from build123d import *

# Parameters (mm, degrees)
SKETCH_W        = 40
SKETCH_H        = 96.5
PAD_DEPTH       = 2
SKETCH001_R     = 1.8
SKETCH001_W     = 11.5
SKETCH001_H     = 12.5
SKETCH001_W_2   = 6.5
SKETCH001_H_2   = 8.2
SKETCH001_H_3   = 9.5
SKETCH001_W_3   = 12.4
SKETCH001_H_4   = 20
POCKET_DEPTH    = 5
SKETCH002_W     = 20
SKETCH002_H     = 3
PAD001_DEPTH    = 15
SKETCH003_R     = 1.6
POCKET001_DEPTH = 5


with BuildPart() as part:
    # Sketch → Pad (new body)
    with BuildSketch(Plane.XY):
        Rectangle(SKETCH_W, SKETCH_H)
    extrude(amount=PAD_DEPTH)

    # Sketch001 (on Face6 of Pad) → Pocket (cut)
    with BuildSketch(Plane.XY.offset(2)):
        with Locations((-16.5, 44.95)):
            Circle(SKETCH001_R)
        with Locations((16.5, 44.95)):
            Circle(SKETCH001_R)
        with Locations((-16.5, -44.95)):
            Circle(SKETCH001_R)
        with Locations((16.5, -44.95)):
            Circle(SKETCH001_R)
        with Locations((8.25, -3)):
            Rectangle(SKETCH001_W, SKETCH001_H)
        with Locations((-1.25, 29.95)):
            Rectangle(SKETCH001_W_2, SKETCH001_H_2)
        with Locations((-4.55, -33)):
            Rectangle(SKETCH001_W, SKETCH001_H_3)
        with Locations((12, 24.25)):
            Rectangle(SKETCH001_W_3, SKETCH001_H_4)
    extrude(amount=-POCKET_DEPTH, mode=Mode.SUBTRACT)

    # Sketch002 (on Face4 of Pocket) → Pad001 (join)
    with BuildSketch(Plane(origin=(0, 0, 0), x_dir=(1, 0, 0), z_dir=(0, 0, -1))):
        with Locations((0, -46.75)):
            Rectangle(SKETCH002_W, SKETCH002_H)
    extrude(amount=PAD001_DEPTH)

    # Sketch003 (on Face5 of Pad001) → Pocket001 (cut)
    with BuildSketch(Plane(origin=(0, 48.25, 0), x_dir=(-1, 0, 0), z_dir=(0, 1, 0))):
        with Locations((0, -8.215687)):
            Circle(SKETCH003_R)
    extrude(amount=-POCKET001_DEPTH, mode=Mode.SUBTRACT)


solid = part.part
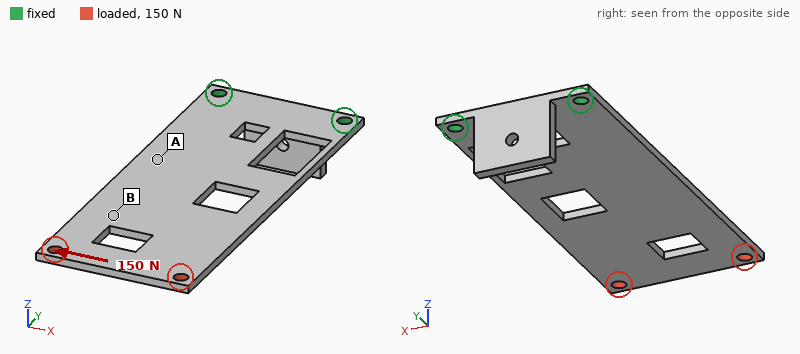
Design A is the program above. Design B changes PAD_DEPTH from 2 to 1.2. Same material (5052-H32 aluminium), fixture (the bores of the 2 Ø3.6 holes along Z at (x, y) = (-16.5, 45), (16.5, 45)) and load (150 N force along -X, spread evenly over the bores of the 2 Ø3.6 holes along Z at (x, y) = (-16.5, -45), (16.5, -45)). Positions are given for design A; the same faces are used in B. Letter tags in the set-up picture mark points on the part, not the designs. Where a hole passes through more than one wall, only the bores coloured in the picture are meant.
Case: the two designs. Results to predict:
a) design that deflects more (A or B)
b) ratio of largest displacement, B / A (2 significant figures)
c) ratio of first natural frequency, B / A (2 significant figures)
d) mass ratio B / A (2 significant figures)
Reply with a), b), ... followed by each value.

a) B
b) 1.7
c) 0.61
d) 0.65
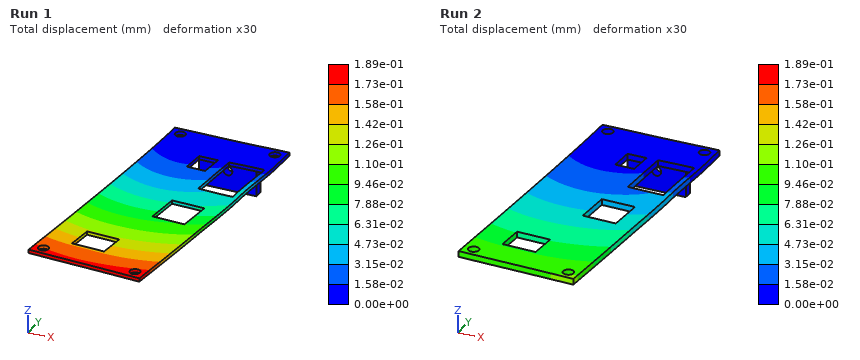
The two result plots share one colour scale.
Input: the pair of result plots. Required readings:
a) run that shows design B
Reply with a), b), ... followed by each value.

a) Run 1
